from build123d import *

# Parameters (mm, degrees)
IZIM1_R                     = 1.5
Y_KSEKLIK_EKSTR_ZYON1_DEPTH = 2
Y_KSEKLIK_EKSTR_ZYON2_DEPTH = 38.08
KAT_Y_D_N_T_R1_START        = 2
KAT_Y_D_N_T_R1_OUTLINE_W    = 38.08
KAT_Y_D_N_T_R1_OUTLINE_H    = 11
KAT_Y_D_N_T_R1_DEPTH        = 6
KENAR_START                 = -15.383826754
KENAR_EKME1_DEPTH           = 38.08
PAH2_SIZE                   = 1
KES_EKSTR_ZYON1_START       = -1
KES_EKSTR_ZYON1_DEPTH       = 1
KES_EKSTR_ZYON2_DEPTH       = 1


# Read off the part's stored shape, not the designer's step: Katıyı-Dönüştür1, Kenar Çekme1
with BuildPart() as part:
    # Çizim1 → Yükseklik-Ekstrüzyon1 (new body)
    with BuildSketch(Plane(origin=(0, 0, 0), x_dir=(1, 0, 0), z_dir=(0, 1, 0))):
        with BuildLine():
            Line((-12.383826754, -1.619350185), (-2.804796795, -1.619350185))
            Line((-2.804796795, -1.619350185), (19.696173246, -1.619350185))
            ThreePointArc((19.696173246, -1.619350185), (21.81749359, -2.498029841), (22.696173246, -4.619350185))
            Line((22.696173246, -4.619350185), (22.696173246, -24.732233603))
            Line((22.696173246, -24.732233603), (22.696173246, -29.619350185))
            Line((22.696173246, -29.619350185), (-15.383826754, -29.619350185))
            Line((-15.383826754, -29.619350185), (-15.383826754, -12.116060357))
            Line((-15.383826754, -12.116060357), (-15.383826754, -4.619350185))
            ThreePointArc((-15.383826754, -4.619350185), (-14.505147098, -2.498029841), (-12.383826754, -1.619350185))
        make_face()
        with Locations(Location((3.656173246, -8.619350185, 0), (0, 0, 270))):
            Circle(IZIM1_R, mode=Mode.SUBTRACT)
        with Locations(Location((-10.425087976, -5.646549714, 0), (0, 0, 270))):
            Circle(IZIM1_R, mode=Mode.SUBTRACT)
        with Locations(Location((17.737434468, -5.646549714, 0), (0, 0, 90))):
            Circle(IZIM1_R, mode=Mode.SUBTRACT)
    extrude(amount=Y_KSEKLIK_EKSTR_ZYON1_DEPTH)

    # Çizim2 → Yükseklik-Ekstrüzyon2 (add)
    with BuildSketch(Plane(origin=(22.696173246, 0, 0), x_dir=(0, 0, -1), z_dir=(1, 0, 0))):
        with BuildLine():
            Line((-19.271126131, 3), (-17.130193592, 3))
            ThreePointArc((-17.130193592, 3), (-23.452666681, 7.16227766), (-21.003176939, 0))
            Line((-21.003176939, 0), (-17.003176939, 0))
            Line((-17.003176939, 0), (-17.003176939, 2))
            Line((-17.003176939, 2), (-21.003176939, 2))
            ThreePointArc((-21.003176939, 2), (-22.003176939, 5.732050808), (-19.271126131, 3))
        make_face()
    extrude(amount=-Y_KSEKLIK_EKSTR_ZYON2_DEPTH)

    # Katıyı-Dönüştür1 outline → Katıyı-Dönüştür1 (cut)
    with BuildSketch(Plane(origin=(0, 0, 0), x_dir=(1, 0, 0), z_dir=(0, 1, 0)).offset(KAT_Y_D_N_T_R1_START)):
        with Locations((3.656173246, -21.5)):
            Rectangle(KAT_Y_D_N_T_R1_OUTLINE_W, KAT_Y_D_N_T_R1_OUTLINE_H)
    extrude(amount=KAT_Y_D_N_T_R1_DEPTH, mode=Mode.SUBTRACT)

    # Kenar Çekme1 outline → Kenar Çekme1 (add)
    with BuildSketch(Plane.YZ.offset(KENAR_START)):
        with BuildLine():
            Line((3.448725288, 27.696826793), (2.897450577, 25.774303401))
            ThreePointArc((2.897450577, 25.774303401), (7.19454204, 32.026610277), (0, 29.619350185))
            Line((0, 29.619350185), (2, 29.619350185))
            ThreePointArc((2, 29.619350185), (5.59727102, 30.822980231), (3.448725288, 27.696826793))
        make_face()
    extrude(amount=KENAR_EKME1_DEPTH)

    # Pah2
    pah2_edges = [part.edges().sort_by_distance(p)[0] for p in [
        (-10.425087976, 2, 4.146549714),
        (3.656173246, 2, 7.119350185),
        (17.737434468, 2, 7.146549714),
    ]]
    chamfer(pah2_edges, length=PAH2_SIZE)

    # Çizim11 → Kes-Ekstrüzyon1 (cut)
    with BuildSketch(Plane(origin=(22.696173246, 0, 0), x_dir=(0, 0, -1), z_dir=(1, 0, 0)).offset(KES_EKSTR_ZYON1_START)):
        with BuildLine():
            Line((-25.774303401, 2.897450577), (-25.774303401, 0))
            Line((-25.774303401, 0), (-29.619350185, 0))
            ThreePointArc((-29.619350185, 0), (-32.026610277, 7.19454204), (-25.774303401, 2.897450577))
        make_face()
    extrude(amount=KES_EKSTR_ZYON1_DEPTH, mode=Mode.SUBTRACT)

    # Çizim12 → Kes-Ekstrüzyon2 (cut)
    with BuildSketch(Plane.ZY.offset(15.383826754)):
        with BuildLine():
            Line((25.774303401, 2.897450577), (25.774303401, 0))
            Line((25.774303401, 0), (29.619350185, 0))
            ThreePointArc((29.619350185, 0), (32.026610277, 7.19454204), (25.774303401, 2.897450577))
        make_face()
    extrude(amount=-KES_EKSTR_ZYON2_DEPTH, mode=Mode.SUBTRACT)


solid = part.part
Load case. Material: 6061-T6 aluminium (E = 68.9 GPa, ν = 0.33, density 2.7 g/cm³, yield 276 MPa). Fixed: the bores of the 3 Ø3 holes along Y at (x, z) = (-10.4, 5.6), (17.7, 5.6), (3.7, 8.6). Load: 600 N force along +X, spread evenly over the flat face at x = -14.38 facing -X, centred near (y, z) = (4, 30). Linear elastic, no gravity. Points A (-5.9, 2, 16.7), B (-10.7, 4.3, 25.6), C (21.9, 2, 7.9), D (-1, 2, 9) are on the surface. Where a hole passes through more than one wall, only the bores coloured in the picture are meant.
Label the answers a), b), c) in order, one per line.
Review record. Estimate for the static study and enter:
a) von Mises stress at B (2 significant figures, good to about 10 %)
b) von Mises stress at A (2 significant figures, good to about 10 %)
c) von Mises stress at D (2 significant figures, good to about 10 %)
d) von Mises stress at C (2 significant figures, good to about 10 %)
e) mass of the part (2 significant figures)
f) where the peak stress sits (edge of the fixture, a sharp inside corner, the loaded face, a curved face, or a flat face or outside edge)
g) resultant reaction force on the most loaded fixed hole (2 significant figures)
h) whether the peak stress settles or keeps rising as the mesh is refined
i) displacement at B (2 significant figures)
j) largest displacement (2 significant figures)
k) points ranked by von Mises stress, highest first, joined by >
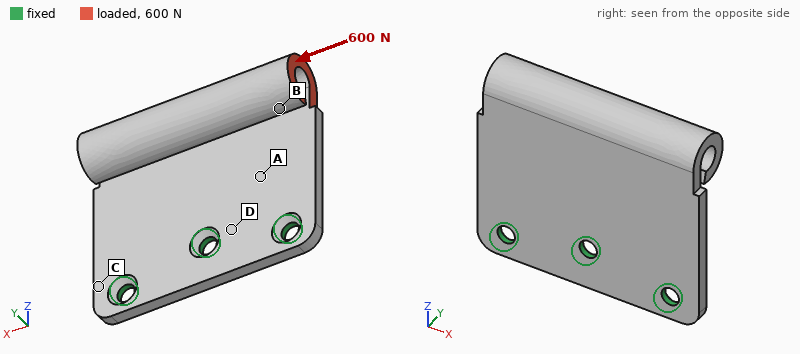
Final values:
a) 20 MPa
b) 57 MPa
c) 31 MPa
d) 41 MPa
e) 8.5 g
f) edge of the fixture
g) 490 N
h) keeps rising
i) 0.14 mm
j) 0.21 mm
k) A > C > D > B
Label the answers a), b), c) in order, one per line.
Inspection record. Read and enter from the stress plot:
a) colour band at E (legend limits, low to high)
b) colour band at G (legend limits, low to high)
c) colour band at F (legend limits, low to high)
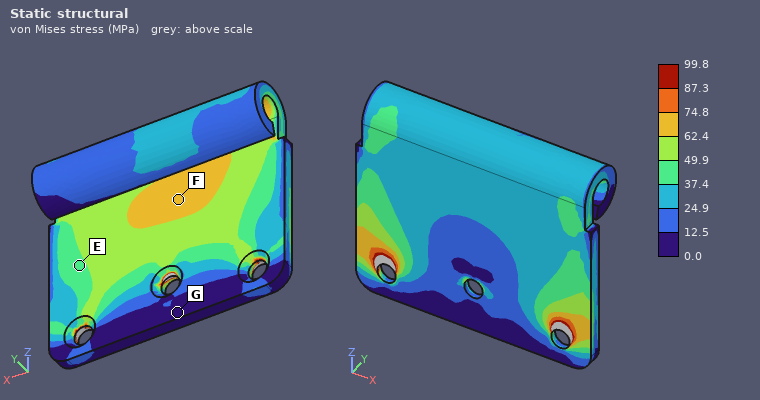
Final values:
a) 37.4 to 49.9 MPa
b) 0.0 to 12.5 MPa
c) 62.4 to 74.8 MPa
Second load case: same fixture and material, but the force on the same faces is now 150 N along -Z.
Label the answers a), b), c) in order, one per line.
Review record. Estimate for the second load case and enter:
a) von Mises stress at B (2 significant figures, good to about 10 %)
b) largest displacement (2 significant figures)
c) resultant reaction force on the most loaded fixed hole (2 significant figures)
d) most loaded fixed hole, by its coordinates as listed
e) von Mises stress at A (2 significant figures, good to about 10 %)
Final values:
a) 11 MPa
b) 0.13 mm
c) 150 N
d) (-10.4, 5.6)
e) 22 MPa
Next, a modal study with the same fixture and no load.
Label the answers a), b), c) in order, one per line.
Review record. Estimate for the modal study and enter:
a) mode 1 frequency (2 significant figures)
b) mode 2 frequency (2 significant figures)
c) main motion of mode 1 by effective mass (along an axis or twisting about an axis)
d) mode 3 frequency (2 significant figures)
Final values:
a) 1500 Hz
b) 2900 Hz
c) along Y
d) 7700 Hz
